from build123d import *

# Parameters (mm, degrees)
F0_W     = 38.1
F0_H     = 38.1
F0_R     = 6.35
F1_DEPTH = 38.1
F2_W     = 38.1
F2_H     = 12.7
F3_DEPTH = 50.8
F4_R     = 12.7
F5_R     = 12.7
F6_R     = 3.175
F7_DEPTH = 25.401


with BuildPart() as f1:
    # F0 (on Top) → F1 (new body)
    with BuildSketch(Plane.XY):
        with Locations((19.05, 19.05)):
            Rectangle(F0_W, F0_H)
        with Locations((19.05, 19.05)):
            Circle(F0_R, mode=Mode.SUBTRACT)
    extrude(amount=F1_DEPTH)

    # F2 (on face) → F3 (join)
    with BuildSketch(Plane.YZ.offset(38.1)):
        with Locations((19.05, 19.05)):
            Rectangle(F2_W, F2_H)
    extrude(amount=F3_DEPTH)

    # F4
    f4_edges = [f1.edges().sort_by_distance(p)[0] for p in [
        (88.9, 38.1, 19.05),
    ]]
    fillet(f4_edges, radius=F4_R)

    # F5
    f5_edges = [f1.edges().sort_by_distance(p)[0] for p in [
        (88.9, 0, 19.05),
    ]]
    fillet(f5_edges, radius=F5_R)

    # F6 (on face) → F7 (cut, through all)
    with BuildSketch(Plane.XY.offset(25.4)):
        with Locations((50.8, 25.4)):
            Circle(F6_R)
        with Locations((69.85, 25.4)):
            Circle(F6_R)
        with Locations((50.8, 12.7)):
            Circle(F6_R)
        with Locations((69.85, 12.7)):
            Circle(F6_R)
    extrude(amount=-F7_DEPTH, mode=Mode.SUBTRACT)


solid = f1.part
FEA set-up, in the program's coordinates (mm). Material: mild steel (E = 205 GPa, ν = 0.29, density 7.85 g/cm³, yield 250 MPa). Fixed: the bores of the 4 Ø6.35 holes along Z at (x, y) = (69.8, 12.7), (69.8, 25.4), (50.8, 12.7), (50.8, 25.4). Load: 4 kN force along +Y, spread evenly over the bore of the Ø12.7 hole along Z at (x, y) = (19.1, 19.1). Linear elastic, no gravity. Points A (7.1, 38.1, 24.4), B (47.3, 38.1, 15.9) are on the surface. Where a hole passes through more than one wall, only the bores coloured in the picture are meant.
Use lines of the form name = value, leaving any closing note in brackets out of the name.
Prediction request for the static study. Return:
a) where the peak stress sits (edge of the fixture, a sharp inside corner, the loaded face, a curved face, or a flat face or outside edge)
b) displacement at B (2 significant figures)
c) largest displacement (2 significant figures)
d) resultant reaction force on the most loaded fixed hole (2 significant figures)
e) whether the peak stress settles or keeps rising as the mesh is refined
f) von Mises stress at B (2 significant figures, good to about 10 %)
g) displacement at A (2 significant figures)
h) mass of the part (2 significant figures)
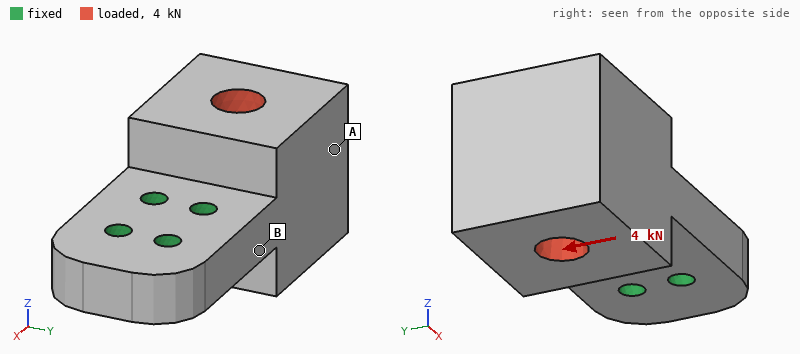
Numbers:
where the peak stress sits = edge of the fixture
displacement at B = 2.6 µm
largest displacement = 13 µm
resultant reaction force on the most loaded fixed hole = 5.1 kN
whether the peak stress settles or keeps rising as the mesh is refined = keeps rising
von Mises stress at B = 31 MPa
displacement at A = 12 µm
mass of the part = 570 g
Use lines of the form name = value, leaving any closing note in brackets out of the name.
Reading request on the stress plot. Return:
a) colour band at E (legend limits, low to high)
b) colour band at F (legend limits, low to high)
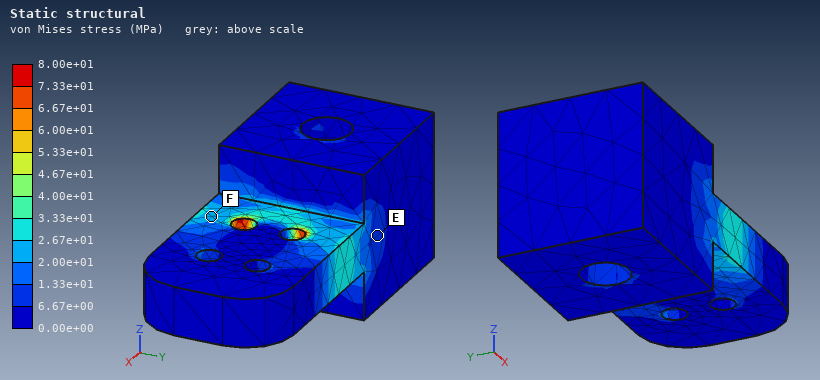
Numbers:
colour band at E = 6.67e+00 to 1.33e+01 MPa
colour band at F = 2.00e+01 to 2.67e+01 MPa
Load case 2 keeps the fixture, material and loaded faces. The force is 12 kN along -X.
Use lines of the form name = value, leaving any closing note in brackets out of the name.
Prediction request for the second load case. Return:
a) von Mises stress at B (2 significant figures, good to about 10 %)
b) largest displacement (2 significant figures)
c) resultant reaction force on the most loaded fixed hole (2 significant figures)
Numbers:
von Mises stress at B = 13 MPa
largest displacement = 4.0 µm
resultant reaction force on the most loaded fixed hole = 5.4 kN
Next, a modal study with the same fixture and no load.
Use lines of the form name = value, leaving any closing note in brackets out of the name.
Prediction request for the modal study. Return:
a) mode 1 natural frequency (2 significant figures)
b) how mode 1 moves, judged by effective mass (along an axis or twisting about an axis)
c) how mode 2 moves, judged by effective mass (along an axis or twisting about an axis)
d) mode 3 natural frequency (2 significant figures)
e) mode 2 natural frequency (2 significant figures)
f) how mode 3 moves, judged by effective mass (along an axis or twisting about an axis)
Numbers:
mode 1 natural frequency = 2500 Hz
how mode 1 moves, judged by effective mass = along Z
how mode 2 moves, judged by effective mass = along Y
mode 3 natural frequency = 6600 Hz
mode 2 natural frequency = 5000 Hz
how mode 3 moves, judged by effective mass = twisting about X
